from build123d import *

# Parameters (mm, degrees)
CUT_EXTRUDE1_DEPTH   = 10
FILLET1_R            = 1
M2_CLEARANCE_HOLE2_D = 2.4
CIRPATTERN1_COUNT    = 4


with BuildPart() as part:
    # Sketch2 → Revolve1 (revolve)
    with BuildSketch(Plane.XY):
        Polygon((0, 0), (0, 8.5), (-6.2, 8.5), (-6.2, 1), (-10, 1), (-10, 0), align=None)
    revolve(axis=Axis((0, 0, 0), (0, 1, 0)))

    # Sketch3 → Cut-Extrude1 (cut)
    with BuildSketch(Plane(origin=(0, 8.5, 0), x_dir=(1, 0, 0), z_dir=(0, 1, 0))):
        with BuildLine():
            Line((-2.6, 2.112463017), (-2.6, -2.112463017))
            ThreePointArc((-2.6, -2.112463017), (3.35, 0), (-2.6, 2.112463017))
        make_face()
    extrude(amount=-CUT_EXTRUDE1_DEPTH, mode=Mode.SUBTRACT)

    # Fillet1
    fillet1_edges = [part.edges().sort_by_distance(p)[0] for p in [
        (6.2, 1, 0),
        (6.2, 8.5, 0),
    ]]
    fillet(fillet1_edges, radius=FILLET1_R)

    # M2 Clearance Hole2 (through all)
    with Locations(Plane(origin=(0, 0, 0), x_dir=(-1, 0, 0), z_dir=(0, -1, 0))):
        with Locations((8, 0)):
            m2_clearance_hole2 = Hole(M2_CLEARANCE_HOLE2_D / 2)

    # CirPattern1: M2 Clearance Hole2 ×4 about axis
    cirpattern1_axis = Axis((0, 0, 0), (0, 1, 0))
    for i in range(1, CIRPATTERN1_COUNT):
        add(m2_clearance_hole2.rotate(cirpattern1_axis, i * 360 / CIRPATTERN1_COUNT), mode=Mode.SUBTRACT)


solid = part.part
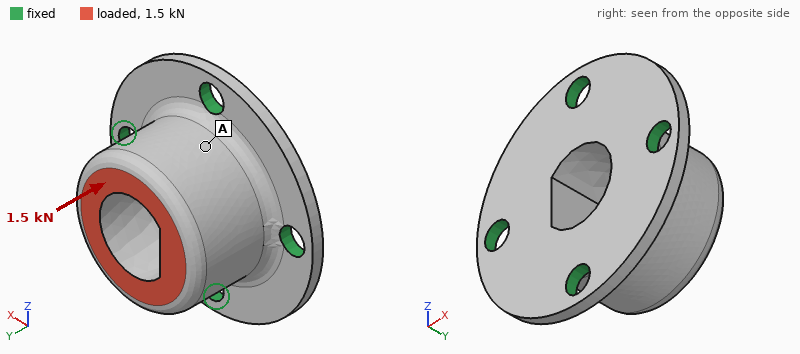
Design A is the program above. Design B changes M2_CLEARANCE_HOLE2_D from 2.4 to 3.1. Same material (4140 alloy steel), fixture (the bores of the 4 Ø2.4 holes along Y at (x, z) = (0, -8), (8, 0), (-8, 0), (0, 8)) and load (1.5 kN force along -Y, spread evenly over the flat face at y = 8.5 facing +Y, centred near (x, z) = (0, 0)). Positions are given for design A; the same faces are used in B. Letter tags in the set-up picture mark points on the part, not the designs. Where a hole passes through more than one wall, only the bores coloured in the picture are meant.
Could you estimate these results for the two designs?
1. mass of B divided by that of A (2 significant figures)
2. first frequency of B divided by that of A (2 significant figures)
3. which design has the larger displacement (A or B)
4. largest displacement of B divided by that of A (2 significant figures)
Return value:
0.99
1.2
A
0.72
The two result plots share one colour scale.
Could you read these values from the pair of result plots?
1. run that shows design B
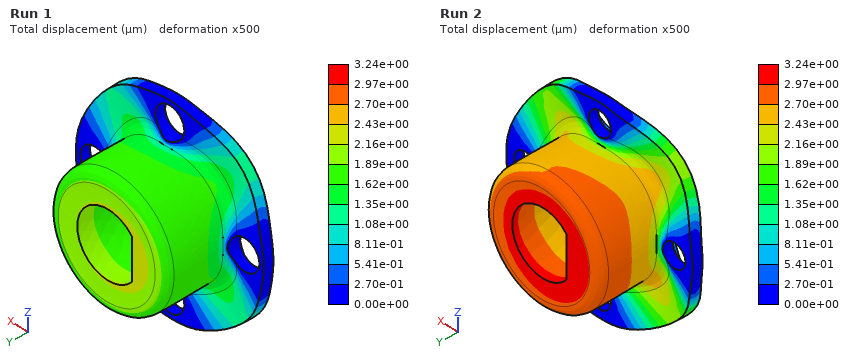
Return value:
Run 1
